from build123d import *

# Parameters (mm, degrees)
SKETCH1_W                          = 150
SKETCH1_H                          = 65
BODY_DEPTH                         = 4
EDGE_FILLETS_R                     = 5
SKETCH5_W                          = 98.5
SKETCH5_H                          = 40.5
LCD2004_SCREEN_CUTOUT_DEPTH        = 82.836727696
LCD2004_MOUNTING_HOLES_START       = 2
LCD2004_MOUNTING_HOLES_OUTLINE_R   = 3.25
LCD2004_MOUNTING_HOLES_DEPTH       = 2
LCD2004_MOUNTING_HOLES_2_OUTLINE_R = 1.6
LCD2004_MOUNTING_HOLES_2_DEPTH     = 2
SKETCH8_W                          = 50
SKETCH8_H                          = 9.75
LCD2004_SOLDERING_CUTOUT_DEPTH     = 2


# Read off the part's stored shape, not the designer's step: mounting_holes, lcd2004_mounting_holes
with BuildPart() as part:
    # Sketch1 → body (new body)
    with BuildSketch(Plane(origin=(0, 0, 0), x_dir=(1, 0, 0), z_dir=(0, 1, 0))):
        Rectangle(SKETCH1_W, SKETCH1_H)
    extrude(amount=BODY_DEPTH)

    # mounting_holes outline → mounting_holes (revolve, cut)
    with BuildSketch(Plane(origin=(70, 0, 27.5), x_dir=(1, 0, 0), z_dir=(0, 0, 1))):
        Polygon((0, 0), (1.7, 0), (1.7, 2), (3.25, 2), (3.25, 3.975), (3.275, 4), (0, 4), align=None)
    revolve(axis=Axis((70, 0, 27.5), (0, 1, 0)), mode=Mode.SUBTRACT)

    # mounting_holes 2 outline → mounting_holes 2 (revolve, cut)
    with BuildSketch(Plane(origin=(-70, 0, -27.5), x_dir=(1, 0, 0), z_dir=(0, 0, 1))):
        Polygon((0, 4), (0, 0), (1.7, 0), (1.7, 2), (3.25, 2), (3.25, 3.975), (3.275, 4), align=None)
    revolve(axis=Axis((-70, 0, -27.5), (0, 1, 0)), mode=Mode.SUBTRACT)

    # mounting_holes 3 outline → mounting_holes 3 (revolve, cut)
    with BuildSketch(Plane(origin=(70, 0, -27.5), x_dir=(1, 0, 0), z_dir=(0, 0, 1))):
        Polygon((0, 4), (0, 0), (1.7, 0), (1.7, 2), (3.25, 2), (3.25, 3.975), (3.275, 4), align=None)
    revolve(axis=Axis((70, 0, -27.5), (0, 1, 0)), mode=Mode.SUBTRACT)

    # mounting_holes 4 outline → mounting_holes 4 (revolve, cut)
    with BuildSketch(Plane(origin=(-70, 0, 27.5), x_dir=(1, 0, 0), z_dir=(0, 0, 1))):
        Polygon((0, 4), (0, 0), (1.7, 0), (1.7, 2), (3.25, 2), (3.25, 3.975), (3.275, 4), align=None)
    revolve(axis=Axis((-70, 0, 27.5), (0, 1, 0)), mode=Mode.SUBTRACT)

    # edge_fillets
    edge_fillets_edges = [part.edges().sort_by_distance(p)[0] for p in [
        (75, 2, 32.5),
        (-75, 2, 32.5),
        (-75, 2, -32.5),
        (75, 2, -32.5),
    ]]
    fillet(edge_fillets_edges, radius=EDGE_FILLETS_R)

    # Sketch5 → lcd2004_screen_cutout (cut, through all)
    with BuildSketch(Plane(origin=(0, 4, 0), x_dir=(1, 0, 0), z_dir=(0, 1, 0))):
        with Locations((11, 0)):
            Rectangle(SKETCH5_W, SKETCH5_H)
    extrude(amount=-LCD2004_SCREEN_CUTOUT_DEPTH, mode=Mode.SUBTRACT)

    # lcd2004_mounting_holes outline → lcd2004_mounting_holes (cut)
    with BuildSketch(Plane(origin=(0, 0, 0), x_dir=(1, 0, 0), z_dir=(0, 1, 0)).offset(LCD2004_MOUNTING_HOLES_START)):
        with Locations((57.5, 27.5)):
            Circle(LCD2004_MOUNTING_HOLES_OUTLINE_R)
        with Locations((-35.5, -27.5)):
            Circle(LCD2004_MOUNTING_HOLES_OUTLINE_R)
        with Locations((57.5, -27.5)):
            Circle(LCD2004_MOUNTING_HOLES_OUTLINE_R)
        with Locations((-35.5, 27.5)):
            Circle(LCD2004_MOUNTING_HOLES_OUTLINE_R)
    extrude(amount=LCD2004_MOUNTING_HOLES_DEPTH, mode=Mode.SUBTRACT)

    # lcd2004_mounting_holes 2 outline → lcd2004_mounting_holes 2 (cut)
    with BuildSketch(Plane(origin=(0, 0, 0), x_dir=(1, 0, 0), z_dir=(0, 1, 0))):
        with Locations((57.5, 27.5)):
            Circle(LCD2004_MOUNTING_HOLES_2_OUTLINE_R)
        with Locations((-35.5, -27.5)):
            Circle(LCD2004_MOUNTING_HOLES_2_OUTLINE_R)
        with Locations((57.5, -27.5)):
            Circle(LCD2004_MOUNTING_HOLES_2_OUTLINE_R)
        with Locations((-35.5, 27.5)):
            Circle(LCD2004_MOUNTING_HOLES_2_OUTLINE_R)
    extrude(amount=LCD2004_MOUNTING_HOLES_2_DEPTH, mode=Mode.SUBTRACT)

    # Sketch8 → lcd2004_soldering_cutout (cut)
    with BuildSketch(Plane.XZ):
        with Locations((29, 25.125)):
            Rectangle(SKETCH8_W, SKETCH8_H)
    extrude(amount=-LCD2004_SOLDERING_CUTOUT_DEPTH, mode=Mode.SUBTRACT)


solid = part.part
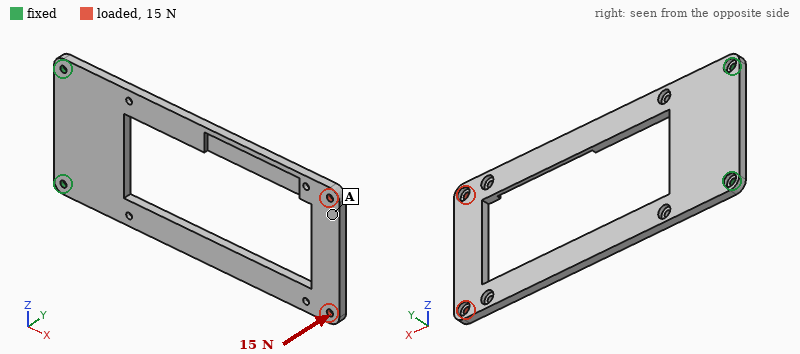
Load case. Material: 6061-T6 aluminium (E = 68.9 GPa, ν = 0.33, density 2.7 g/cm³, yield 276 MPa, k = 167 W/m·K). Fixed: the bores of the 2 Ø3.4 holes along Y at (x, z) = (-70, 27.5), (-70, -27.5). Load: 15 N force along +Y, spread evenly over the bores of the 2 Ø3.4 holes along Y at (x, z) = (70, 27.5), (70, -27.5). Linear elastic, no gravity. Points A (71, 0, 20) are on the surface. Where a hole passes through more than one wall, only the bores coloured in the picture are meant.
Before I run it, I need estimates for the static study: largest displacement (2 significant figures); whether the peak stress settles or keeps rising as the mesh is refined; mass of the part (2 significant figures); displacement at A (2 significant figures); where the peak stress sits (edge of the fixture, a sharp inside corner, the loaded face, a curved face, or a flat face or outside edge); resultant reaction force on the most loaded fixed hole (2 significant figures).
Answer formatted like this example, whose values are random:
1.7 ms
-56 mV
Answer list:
1.7 mm
keeps rising
58 g
1.6 mm
edge of the fixture
7.6 N
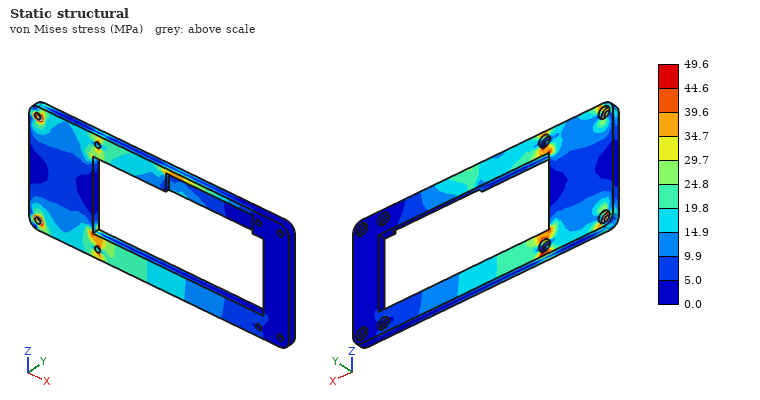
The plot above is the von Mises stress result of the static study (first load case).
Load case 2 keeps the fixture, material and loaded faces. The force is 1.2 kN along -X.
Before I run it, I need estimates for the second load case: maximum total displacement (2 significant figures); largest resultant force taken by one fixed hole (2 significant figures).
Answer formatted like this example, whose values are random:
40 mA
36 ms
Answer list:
1.6 mm
600 N
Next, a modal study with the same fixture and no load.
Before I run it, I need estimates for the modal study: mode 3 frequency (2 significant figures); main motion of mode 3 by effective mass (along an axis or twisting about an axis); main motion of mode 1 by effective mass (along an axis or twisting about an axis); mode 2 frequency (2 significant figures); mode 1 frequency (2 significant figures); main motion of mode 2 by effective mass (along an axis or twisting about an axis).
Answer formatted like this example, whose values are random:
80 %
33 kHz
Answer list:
780 Hz
along Y
along Y
470 Hz
130 Hz
twisting about X
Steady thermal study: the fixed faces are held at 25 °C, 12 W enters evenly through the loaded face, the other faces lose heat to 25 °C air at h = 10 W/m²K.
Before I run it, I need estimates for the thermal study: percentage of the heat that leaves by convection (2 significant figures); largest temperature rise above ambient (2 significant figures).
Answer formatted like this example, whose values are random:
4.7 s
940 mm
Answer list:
40 %
84 K
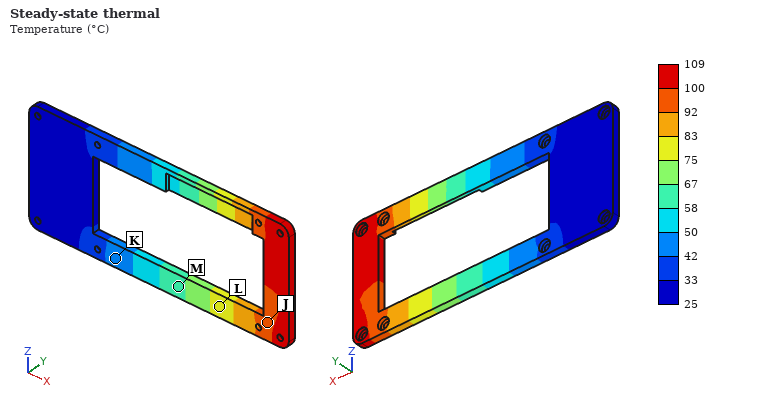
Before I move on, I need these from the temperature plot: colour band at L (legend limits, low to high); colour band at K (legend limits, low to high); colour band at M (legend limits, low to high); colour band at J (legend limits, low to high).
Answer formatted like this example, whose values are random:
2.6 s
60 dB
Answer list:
75 to 83 °C
42 to 50 °C
58 to 67 °C
92 to 100 °C
